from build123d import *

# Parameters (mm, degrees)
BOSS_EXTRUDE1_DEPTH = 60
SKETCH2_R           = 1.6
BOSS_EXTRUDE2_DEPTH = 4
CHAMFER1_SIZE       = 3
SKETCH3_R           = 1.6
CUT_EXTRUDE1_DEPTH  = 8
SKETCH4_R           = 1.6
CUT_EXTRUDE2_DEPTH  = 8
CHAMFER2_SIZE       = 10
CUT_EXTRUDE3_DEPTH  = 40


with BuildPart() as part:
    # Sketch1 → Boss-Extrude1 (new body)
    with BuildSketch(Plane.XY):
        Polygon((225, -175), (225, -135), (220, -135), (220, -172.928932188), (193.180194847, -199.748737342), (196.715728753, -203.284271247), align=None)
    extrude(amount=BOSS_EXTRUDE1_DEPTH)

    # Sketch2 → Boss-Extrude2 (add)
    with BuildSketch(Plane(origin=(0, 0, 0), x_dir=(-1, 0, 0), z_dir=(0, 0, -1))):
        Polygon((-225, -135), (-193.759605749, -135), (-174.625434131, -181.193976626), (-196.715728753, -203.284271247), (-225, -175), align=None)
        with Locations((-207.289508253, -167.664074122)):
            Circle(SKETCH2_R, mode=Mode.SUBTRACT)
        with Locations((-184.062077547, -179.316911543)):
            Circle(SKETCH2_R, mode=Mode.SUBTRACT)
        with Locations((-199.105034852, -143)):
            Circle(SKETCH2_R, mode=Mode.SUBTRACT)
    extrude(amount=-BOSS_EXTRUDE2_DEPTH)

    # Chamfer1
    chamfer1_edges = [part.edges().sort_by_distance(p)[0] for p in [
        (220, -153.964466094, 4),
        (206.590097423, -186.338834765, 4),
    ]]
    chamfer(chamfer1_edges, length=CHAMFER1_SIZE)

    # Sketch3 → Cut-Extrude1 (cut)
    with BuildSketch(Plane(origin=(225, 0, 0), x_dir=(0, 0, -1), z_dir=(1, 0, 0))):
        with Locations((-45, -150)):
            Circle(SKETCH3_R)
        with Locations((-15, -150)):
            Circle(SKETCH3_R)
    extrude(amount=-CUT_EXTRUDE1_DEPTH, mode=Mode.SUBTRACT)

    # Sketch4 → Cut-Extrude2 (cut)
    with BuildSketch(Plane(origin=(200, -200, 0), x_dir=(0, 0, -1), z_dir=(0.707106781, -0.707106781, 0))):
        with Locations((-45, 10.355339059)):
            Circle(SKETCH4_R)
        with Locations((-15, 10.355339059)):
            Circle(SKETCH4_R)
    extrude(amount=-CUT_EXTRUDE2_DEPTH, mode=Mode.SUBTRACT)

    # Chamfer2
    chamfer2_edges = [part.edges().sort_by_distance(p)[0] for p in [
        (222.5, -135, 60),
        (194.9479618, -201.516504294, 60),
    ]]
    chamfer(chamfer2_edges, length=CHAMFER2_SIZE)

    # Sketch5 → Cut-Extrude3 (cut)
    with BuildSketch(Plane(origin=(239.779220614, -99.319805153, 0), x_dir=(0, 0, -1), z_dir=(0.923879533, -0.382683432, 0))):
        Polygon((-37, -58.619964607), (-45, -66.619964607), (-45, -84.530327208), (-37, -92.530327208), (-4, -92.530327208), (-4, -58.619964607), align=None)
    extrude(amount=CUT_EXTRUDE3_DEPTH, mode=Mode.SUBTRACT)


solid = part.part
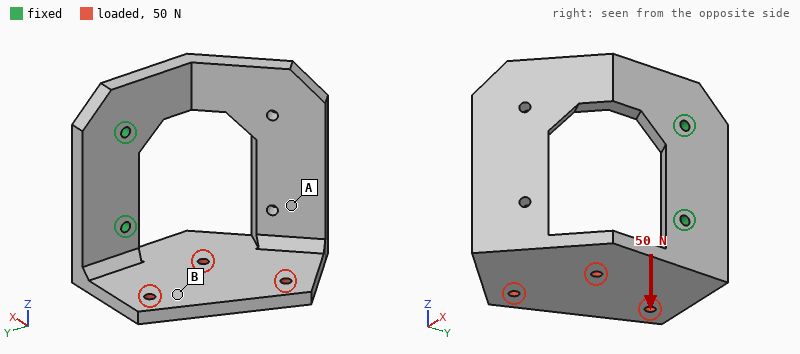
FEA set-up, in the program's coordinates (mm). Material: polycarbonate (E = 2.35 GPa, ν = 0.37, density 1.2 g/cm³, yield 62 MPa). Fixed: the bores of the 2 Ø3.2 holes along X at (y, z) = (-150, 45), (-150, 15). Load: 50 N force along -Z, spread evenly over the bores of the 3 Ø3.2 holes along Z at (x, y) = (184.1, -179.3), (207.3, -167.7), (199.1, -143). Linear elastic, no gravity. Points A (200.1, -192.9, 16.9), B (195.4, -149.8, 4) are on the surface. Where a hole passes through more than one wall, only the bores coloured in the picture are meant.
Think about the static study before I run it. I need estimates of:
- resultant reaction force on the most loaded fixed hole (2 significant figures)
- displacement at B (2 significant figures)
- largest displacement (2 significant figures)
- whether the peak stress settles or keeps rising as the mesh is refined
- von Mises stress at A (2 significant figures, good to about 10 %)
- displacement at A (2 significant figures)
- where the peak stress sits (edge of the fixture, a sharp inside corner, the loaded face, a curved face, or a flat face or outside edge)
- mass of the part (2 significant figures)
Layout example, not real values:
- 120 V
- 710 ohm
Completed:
- 37 N
- 0.68 mm
- 1.2 mm
- keeps rising
- 3.4 MPa
- 0.30 mm
- edge of the fixture
- 28 g
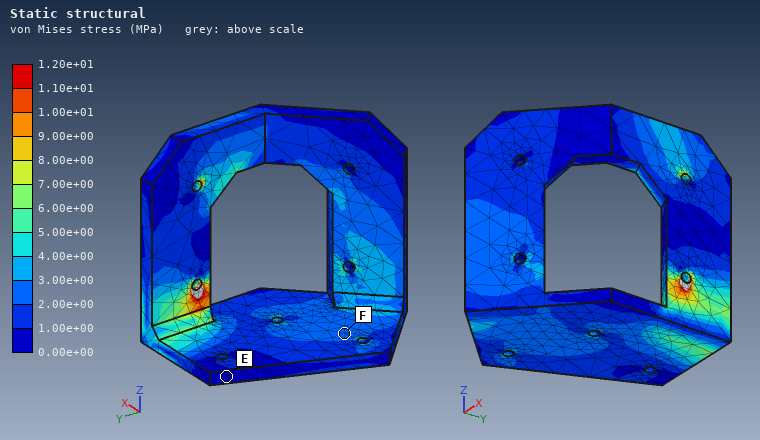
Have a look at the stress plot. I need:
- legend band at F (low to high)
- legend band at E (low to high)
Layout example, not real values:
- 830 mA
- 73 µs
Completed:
- 2.00e+00 to 3.00e+00 MPa
- 0.00e+00 to 1.00e+00 MPa
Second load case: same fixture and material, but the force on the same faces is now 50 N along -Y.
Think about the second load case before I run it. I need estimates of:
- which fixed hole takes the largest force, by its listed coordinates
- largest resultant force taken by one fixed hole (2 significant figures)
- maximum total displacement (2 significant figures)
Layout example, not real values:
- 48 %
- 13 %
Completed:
- (-150, 15)
- 70 N
- 1.2 mm
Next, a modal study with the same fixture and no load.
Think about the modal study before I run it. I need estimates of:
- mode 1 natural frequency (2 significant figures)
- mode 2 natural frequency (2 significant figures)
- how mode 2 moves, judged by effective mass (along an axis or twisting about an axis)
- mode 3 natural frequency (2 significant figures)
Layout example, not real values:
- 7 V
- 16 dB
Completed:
- 250 Hz
- 380 Hz
- along Z
- 740 Hz
